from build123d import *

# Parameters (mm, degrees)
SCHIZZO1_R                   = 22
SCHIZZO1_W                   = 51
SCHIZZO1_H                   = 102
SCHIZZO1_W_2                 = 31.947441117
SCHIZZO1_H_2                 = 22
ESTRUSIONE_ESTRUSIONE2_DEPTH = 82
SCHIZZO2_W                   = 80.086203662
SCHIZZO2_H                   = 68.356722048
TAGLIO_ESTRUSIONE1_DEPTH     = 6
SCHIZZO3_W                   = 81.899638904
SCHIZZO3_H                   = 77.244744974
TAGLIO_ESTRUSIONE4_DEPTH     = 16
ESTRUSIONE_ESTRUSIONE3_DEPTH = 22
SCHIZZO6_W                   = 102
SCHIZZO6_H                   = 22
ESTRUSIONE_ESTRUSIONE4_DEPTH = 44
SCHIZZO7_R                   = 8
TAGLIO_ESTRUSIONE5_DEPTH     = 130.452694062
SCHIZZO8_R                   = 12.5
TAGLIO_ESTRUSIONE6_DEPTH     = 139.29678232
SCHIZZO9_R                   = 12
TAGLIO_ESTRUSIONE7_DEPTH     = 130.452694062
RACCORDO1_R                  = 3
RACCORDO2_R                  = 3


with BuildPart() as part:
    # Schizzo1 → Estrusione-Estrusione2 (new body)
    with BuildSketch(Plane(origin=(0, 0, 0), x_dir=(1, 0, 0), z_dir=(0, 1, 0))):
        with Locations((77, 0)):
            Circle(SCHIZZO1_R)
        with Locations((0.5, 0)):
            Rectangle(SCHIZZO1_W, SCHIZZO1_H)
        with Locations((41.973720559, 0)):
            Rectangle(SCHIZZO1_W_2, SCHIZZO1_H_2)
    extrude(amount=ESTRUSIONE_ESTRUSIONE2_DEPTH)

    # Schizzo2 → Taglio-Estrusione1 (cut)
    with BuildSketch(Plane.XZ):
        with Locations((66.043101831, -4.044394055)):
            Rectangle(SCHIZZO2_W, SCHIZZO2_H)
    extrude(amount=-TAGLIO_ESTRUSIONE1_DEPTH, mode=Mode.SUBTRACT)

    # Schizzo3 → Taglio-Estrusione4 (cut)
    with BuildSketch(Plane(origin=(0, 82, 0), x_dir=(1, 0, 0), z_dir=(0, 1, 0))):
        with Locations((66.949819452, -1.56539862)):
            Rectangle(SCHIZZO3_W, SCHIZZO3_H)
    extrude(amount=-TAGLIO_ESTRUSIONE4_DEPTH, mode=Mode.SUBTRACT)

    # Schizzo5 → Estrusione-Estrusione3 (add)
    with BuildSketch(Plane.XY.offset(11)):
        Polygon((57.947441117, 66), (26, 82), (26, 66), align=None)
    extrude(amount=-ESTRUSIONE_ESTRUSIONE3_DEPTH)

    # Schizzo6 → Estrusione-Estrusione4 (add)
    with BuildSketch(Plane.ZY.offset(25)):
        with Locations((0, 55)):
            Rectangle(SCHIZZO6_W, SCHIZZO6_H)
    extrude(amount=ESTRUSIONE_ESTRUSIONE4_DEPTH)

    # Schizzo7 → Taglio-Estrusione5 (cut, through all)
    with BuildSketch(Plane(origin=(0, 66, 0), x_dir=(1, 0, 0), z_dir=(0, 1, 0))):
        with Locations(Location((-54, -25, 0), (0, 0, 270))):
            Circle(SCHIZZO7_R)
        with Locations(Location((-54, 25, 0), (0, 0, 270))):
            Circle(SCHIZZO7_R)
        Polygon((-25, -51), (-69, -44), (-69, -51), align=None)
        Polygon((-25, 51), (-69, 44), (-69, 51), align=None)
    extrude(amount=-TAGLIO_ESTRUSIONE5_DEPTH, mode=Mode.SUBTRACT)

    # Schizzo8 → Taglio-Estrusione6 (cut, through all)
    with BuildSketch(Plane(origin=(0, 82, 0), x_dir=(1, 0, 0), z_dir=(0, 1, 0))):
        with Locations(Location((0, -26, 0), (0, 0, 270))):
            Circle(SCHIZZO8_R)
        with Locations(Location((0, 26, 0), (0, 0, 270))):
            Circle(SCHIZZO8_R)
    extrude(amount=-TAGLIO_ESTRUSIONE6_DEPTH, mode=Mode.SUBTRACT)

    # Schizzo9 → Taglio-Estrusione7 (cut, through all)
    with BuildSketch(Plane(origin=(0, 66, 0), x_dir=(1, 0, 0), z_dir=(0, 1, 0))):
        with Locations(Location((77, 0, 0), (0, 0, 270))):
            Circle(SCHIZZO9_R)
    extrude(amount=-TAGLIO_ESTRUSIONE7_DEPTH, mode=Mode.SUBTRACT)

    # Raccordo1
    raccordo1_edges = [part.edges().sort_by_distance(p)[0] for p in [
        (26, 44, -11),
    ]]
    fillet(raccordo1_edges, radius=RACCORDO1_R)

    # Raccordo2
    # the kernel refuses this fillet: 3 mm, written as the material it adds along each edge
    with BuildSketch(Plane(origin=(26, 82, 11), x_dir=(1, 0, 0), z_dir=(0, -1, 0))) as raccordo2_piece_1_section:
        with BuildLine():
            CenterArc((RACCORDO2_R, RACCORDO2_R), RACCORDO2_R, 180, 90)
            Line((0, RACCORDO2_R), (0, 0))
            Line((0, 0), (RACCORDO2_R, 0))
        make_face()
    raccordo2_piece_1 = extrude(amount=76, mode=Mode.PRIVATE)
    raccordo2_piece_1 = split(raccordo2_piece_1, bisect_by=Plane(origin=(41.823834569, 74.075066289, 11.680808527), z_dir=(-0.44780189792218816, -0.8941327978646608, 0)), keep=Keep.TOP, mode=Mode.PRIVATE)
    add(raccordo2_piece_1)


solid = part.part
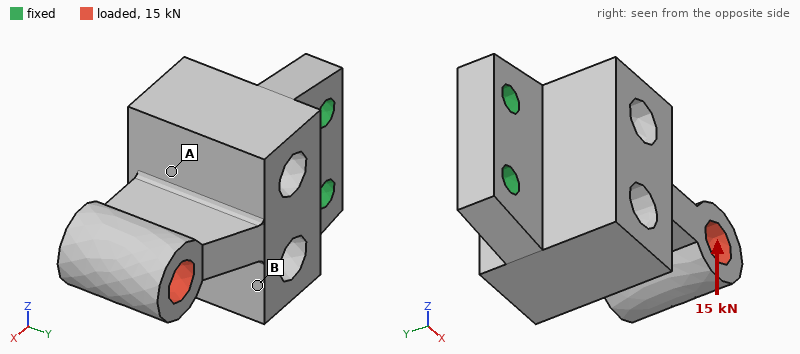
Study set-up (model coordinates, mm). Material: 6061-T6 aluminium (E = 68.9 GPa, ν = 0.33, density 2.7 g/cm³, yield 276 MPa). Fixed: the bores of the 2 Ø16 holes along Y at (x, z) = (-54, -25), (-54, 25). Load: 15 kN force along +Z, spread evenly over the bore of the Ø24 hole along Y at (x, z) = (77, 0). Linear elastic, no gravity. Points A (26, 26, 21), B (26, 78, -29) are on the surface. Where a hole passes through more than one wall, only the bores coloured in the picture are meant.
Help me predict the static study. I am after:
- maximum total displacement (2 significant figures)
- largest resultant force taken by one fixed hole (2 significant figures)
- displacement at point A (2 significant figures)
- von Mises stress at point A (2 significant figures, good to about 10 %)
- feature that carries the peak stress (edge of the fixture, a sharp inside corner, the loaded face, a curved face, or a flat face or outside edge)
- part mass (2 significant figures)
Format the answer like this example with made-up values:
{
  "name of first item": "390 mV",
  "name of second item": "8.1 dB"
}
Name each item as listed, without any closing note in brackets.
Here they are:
{
  "maximum total displacement": "0.61 mm",
  "largest resultant force taken by one fixed hole": "32 kN",
  "displacement at point A": "0.092 mm",
  "von Mises stress at point A": "30 MPa",
  "feature that carries the peak stress": "a curved face",
  "part mass": "1.5 kg"
}
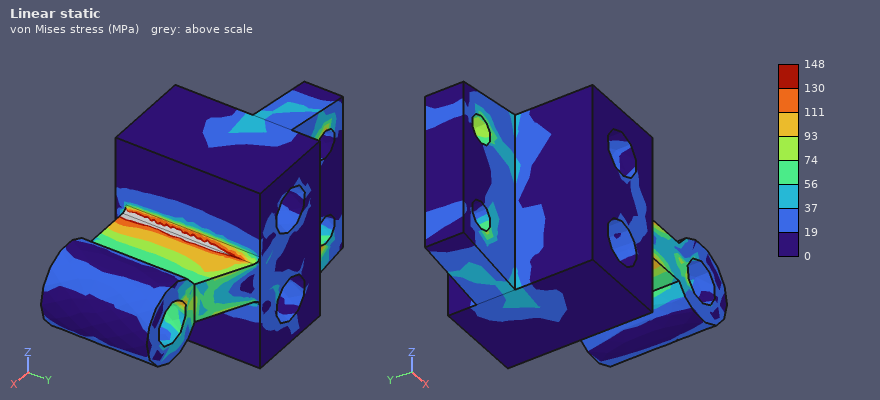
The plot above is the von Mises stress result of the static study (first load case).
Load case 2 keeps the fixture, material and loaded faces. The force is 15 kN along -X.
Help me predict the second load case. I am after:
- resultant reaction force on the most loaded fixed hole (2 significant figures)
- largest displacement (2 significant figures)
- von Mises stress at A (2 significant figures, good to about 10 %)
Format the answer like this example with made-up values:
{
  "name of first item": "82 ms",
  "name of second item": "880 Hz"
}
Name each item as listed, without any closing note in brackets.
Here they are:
{
  "resultant reaction force on the most loaded fixed hole": "7.6 kN",
  "largest displacement": "0.25 mm",
  "von Mises stress at A": "4.6 MPa"
}
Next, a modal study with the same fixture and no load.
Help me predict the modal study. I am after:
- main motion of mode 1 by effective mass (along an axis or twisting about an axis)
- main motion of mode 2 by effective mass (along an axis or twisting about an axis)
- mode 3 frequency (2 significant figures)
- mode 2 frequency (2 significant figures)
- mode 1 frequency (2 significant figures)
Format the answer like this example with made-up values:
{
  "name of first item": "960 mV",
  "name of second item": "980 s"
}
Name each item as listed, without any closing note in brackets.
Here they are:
{
  "main motion of mode 1 by effective mass": "along Y",
  "main motion of mode 2 by effective mass": "along Z",
  "mode 3 frequency": "3100 Hz",
  "mode 2 frequency": "1900 Hz",
  "mode 1 frequency": "900 Hz"
}
